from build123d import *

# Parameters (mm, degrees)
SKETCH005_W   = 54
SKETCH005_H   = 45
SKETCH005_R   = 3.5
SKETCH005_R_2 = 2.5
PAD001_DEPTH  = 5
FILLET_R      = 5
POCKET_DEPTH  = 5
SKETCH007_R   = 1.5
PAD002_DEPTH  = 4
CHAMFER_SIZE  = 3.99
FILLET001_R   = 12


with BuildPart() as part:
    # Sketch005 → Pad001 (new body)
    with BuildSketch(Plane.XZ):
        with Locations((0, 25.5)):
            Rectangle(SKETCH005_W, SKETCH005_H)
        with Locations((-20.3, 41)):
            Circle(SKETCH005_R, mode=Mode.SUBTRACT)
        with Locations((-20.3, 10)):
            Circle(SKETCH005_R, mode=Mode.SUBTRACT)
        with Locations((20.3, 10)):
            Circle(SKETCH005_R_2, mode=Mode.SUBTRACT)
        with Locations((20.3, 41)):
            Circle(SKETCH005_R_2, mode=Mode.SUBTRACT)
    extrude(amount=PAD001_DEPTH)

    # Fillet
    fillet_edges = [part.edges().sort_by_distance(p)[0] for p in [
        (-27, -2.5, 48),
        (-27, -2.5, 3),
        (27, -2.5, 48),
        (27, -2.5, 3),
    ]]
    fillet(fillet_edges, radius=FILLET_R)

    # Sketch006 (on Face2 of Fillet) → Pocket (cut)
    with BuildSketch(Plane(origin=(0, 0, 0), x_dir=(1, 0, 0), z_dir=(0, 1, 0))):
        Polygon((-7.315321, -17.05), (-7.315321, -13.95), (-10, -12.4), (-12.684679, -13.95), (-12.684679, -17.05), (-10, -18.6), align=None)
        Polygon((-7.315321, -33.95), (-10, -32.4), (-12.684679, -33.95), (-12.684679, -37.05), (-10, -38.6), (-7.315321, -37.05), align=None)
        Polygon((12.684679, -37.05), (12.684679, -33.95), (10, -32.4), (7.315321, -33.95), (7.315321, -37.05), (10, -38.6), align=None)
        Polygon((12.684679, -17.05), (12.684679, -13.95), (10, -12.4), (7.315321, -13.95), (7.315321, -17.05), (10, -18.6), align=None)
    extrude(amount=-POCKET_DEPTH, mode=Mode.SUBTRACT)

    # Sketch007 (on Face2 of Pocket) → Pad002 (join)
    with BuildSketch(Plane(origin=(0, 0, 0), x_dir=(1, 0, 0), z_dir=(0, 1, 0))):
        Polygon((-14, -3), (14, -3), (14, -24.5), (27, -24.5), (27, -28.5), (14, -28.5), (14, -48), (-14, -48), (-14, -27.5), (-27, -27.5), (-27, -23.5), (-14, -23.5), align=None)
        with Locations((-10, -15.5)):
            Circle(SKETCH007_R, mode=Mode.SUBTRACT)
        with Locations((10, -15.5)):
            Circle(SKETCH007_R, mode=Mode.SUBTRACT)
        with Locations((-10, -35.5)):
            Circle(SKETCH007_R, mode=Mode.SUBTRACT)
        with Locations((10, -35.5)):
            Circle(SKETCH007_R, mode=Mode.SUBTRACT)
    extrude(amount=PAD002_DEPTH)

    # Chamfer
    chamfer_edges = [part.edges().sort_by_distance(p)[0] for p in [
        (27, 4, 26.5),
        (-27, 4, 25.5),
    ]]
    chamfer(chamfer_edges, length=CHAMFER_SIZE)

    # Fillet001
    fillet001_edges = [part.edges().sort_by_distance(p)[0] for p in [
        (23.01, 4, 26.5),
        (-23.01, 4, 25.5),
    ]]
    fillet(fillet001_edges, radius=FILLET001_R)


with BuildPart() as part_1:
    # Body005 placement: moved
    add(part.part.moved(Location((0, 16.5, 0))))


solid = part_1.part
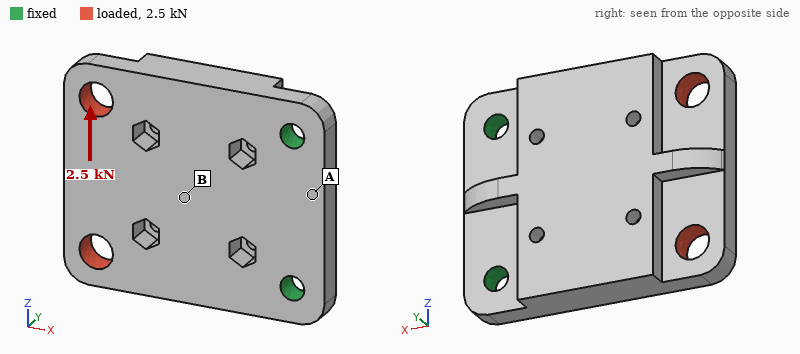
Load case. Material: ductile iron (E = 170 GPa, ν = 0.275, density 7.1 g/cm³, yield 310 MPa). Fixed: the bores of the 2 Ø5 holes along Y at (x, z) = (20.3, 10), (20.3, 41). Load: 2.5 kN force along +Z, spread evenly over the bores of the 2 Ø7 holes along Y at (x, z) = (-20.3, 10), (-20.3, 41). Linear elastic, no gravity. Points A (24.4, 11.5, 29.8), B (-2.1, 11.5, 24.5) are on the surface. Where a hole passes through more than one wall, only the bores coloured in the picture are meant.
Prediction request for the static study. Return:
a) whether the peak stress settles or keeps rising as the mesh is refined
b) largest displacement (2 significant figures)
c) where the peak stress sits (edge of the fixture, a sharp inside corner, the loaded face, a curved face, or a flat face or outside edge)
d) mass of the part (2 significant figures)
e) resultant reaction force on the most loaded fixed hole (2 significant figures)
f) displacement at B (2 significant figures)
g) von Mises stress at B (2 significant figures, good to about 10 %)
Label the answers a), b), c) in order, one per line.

a) keeps rising
b) 26 µm
c) edge of the fixture
d) 120 g
e) 3.2 kN
f) 9.2 µm
g) 26 MPa
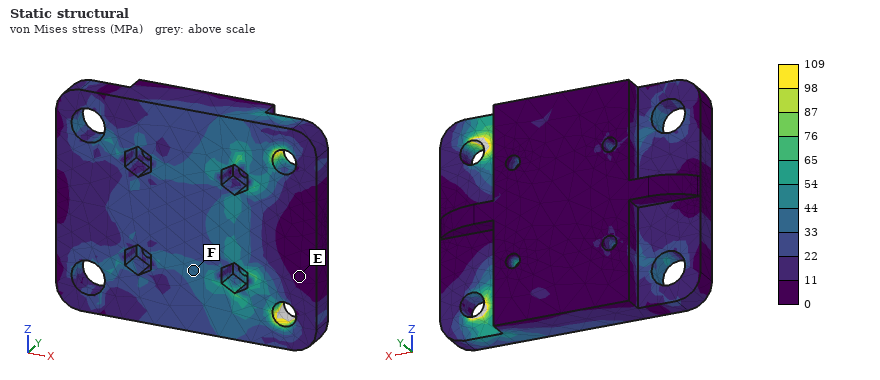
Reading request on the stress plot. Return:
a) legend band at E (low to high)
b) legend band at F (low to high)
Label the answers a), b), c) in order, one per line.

a) 0 to 11 MPa
b) 33 to 44 MPa
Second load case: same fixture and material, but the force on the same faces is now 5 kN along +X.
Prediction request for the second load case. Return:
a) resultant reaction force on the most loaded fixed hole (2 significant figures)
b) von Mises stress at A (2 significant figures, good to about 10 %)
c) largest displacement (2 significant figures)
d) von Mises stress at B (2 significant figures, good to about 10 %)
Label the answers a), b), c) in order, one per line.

a) 2.5 kN
b) 7.2 MPa
c) 21 µm
d) 25 MPa
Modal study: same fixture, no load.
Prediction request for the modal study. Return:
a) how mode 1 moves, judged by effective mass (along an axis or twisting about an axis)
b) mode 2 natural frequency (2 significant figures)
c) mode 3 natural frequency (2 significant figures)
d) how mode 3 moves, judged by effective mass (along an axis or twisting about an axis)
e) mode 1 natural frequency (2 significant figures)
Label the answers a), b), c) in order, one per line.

a) along Y
b) 6600 Hz
c) 10000 Hz
d) along Z
e) 2000 Hz
